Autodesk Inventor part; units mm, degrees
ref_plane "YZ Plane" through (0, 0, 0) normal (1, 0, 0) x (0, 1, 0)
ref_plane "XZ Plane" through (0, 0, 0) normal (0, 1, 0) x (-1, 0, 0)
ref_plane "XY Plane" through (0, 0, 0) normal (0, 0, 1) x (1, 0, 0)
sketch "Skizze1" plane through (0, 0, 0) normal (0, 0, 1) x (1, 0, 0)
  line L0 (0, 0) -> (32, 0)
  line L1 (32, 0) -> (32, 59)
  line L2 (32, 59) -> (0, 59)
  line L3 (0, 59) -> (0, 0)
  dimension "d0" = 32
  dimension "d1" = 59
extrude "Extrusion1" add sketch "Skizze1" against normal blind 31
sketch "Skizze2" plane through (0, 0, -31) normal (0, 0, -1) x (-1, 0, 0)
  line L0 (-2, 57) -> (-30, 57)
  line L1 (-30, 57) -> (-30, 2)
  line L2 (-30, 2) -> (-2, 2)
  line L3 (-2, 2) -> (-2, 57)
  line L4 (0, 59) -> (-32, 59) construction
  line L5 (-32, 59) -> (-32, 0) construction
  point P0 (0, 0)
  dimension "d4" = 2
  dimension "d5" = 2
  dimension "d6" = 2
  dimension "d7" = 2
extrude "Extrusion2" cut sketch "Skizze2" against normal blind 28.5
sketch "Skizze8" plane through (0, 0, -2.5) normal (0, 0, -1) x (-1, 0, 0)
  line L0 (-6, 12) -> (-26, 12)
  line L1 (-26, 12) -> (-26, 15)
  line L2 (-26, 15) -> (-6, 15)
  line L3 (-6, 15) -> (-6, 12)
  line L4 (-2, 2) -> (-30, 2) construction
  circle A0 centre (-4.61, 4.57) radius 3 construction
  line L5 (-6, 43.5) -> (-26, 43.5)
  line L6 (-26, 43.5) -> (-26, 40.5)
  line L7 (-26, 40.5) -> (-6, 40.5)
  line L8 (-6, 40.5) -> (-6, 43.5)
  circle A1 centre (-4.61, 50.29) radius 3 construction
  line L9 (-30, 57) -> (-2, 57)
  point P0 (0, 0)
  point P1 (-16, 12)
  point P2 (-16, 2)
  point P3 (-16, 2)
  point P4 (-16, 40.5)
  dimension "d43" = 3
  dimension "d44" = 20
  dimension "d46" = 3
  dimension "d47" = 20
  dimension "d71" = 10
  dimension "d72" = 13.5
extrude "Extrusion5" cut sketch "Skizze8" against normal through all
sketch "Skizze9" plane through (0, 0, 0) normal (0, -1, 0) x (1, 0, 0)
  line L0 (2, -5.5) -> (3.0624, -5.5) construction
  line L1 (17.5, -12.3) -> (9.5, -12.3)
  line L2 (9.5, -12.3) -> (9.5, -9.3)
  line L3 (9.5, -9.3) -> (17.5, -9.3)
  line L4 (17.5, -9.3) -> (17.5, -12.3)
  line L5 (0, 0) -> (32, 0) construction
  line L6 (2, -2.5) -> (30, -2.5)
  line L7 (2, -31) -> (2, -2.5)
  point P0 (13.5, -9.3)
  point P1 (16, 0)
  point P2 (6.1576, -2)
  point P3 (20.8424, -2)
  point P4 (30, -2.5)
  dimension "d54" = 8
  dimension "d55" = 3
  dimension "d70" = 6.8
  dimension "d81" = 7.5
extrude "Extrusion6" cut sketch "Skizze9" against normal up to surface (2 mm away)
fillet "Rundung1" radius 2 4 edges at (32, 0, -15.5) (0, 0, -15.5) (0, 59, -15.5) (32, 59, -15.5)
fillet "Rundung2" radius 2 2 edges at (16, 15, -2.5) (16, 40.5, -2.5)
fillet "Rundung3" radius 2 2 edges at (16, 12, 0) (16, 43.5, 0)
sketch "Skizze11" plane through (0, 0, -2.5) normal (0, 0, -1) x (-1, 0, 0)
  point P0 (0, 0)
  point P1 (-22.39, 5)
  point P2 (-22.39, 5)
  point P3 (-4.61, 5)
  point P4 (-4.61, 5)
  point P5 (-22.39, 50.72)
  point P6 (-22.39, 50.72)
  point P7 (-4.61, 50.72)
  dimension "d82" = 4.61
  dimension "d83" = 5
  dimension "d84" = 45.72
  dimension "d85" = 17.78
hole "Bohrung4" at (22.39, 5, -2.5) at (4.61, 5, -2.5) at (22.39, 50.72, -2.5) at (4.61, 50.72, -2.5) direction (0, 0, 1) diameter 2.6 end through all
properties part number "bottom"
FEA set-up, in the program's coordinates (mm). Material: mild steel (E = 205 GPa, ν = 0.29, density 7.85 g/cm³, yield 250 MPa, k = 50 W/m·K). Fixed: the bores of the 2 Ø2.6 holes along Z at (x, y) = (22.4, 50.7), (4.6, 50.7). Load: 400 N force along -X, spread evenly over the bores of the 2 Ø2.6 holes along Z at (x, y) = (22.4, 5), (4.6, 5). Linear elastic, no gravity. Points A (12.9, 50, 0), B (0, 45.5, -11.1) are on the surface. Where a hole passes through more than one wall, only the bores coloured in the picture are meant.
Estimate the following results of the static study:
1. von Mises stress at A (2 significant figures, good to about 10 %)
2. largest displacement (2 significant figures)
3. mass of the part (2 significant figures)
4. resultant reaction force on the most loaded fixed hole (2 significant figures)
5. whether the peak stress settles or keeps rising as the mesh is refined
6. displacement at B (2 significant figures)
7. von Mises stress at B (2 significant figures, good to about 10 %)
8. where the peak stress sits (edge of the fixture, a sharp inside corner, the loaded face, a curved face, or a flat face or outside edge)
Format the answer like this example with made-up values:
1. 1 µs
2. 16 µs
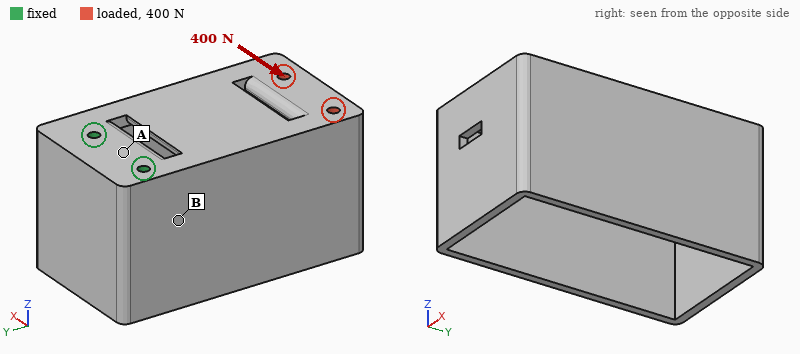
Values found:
1. 22 MPa
2. 26 µm
3. 110 g
4. 950 N
5. keeps rising
6. 4.1 µm
7. 8.3 MPa
8. edge of the fixture
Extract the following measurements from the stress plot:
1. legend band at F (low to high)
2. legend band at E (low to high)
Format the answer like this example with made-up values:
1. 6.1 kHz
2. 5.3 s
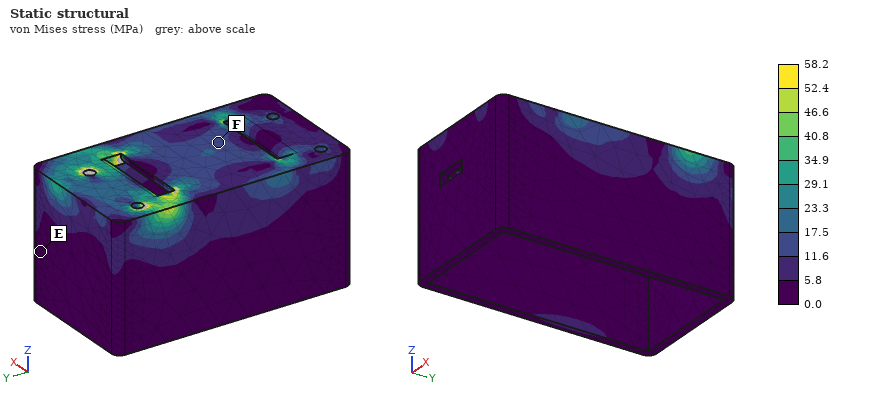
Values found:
1. 11.6 to 17.5 MPa
2. 0.0 to 5.8 MPa
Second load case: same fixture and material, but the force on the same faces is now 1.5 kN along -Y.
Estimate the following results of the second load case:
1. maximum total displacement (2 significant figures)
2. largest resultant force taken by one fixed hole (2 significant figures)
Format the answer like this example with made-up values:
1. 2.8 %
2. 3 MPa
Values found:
1. 13 µm
2. 770 N
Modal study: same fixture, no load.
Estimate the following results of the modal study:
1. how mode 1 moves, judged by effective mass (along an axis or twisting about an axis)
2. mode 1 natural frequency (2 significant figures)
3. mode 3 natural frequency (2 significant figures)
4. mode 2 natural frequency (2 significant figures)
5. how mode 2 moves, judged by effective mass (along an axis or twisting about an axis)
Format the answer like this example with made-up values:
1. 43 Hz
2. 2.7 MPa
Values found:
1. along Z
2. 820 Hz
3. 3300 Hz
4. 1400 Hz
5. along X
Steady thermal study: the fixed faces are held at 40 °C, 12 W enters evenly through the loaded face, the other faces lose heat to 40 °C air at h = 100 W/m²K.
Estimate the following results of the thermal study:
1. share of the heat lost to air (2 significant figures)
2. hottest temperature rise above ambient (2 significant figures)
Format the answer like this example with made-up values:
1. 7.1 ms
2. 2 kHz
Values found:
1. 93 %
2. 41 K
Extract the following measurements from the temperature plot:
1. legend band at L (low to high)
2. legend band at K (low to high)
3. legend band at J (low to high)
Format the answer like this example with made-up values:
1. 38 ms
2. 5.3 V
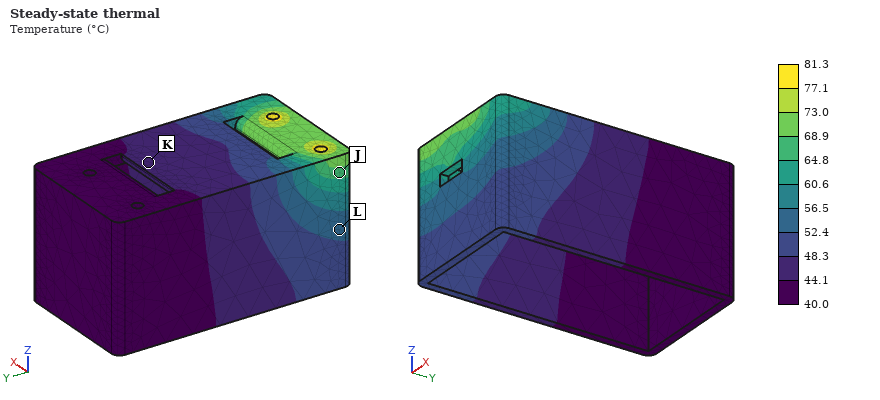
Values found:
1. 52.4 to 56.5 °C
2. 44.1 to 48.3 °C
3. 64.8 to 68.9 °C
